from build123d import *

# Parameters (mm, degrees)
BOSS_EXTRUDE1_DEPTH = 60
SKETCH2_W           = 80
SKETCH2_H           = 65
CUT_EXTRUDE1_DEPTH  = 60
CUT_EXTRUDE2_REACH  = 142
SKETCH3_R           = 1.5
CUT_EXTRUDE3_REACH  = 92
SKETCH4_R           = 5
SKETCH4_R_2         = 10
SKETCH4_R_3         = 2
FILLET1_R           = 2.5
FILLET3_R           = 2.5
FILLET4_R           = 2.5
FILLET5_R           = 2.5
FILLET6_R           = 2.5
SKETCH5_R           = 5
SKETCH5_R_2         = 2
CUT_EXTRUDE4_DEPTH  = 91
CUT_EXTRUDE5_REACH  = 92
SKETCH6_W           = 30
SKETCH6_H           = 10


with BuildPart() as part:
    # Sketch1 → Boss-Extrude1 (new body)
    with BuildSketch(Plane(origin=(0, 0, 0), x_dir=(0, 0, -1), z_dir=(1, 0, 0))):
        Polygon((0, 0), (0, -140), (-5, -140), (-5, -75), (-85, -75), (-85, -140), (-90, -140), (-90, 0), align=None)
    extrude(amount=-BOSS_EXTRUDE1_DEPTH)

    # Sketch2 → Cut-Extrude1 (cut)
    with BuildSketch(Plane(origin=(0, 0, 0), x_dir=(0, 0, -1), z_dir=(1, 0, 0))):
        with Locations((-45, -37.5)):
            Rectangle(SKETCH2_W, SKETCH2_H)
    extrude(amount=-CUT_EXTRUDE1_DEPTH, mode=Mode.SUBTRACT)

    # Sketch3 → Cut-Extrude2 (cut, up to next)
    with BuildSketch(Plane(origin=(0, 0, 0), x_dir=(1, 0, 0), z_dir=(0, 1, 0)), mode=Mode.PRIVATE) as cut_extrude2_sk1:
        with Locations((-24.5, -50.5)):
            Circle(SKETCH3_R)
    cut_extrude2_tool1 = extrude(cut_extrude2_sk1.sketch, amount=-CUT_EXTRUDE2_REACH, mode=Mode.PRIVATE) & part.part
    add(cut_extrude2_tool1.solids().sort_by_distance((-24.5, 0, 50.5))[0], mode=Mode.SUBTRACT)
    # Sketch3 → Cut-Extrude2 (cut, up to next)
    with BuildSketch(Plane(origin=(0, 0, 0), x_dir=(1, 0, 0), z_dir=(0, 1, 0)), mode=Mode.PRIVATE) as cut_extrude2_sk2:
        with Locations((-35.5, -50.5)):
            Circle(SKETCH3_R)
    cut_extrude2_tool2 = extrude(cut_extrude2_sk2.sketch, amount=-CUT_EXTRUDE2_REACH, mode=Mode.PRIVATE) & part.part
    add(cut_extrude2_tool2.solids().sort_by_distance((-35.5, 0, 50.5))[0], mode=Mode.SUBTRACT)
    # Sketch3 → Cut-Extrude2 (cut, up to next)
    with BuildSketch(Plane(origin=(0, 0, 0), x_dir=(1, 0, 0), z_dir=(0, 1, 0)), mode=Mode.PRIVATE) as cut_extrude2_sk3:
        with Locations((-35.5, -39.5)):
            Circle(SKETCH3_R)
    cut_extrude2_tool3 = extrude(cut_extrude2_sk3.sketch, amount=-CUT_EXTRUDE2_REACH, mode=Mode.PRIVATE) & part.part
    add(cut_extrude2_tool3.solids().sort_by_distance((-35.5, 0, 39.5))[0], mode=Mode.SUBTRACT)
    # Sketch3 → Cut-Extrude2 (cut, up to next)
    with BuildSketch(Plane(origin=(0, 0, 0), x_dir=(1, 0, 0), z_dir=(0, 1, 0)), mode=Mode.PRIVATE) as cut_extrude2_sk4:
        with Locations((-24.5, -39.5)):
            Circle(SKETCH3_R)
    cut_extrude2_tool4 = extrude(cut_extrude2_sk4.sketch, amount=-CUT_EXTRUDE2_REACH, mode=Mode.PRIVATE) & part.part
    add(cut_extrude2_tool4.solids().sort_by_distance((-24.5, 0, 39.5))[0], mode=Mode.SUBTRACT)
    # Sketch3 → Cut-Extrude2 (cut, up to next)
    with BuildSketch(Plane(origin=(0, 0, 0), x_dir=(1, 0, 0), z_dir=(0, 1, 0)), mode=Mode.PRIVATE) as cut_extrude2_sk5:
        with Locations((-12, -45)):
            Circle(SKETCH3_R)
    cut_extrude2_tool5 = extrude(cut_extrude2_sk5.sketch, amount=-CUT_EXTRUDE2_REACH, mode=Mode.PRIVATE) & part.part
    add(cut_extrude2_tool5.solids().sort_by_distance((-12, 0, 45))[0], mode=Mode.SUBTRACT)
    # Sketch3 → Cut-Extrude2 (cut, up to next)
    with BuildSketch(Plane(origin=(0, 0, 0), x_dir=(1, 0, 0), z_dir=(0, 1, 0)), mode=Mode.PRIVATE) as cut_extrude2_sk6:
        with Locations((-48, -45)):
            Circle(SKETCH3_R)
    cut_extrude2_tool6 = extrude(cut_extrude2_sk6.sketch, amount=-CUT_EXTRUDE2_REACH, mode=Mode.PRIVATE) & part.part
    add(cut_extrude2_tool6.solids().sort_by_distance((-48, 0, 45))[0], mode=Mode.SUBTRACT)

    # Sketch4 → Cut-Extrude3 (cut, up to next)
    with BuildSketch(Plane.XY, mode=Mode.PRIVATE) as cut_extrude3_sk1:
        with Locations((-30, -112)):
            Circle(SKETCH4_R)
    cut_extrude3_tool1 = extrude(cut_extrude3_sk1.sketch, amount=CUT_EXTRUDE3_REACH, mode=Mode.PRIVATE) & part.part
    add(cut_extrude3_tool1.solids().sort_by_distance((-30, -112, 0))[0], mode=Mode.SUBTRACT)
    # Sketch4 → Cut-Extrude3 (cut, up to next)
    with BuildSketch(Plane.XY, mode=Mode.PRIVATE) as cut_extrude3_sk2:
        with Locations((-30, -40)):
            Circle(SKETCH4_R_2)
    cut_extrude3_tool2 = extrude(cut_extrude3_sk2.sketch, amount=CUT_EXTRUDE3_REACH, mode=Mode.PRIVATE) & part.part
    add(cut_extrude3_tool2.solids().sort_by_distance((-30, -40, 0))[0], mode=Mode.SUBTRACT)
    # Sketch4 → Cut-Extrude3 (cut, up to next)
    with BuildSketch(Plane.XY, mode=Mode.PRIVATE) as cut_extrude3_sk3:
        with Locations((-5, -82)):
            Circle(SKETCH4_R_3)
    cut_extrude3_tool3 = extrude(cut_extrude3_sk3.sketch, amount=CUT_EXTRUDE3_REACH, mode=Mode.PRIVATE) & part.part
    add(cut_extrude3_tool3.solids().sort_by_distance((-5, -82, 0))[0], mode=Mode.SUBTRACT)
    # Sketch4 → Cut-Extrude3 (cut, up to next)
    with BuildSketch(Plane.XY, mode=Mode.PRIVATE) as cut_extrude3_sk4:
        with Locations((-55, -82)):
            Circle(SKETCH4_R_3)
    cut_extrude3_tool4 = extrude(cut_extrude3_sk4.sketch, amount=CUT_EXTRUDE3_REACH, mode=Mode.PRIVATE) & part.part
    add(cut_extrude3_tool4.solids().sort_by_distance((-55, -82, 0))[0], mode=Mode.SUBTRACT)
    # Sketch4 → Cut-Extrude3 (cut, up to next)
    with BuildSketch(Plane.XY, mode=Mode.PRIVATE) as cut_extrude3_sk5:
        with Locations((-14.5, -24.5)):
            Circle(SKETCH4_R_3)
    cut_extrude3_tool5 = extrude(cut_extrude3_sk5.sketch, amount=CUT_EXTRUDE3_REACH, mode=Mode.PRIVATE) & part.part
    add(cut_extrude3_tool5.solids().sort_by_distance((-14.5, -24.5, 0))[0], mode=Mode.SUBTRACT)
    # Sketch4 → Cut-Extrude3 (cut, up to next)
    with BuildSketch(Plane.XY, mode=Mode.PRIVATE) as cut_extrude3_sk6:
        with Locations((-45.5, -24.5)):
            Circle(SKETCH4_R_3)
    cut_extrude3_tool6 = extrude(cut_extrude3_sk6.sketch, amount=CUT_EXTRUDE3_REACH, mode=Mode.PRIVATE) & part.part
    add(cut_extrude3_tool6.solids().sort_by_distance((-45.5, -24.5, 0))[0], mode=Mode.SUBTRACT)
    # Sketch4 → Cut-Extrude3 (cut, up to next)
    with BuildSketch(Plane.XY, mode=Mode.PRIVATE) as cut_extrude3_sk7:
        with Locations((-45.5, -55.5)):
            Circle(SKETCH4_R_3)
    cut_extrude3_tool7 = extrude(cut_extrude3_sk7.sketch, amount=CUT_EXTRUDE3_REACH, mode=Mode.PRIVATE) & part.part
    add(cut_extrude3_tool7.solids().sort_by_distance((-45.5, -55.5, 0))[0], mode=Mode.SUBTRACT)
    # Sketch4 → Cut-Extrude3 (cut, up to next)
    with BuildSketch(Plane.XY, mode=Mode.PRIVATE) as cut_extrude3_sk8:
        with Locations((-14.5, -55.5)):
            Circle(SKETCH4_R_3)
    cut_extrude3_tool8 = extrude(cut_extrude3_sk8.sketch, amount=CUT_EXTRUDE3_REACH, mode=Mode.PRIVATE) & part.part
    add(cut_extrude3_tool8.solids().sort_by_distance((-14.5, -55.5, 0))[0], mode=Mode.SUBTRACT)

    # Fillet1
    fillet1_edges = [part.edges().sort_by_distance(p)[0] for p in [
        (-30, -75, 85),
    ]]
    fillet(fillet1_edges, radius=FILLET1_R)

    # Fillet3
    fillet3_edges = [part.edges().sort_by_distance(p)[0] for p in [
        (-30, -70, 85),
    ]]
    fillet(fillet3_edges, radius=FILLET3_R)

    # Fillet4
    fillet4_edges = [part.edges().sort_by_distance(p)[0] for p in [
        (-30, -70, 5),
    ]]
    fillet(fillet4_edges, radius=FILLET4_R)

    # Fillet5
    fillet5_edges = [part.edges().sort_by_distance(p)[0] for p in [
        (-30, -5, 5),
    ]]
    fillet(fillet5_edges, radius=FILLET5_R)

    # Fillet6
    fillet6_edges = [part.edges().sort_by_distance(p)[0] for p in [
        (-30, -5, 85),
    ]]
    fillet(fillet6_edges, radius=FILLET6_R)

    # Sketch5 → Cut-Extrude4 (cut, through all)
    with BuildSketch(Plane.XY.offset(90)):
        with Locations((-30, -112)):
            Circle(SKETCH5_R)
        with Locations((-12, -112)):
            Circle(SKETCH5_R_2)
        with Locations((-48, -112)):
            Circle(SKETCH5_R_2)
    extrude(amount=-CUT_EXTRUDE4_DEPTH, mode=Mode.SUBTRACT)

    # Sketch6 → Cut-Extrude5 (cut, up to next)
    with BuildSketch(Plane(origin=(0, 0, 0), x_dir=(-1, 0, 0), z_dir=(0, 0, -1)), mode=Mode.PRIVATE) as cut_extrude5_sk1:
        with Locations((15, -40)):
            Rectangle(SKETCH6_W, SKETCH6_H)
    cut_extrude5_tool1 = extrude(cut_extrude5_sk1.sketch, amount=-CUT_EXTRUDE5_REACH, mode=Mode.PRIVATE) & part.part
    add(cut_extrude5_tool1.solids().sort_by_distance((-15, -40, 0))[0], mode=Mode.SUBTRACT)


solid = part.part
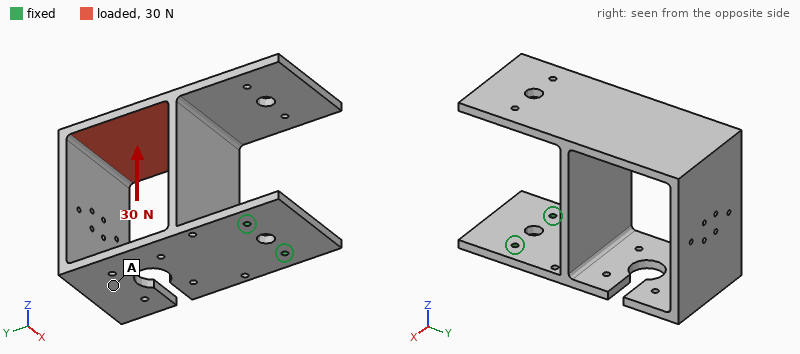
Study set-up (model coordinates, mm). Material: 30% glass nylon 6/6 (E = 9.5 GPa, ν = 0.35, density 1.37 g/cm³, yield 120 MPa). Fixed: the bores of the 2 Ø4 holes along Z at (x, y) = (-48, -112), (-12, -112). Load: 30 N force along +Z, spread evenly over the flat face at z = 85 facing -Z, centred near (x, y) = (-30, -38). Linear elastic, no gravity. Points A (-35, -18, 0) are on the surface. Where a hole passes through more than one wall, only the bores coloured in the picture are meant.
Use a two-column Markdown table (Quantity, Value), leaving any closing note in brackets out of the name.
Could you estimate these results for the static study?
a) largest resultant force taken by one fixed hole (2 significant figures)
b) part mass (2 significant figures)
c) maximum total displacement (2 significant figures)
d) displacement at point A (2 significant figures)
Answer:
| Quantity | Value |
|---|---|
| largest resultant force taken by one fixed hole | 15 N |
| part mass | 180 g |
| maximum total displacement | 1.8 mm |
| displacement at point A | 1.0 mm |
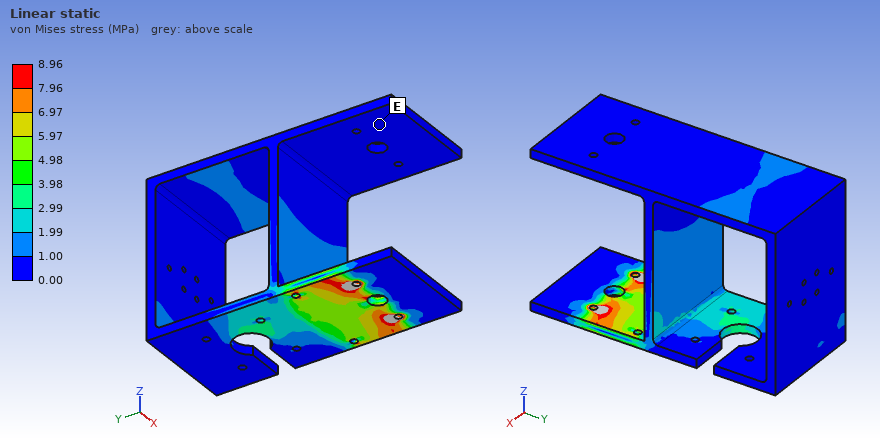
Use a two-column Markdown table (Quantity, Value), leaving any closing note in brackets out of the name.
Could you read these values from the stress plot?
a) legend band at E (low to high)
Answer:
| Quantity | Value |
|---|---|
| legend band at E | 0.00 to 1.00 MPa |
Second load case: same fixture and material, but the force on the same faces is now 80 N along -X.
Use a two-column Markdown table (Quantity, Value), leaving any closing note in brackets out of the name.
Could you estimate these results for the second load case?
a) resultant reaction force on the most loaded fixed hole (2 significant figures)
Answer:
| Quantity | Value |
|---|---|
| resultant reaction force on the most loaded fixed hole | 230 N |
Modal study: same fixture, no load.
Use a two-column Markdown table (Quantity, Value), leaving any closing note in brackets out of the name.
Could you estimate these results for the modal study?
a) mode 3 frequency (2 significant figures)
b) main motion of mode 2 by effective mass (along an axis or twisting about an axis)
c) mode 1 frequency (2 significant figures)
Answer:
| Quantity | Value |
|---|---|
| mode 3 frequency | 250 Hz |
| main motion of mode 2 by effective mass | along X |
| mode 1 frequency | 53 Hz |
